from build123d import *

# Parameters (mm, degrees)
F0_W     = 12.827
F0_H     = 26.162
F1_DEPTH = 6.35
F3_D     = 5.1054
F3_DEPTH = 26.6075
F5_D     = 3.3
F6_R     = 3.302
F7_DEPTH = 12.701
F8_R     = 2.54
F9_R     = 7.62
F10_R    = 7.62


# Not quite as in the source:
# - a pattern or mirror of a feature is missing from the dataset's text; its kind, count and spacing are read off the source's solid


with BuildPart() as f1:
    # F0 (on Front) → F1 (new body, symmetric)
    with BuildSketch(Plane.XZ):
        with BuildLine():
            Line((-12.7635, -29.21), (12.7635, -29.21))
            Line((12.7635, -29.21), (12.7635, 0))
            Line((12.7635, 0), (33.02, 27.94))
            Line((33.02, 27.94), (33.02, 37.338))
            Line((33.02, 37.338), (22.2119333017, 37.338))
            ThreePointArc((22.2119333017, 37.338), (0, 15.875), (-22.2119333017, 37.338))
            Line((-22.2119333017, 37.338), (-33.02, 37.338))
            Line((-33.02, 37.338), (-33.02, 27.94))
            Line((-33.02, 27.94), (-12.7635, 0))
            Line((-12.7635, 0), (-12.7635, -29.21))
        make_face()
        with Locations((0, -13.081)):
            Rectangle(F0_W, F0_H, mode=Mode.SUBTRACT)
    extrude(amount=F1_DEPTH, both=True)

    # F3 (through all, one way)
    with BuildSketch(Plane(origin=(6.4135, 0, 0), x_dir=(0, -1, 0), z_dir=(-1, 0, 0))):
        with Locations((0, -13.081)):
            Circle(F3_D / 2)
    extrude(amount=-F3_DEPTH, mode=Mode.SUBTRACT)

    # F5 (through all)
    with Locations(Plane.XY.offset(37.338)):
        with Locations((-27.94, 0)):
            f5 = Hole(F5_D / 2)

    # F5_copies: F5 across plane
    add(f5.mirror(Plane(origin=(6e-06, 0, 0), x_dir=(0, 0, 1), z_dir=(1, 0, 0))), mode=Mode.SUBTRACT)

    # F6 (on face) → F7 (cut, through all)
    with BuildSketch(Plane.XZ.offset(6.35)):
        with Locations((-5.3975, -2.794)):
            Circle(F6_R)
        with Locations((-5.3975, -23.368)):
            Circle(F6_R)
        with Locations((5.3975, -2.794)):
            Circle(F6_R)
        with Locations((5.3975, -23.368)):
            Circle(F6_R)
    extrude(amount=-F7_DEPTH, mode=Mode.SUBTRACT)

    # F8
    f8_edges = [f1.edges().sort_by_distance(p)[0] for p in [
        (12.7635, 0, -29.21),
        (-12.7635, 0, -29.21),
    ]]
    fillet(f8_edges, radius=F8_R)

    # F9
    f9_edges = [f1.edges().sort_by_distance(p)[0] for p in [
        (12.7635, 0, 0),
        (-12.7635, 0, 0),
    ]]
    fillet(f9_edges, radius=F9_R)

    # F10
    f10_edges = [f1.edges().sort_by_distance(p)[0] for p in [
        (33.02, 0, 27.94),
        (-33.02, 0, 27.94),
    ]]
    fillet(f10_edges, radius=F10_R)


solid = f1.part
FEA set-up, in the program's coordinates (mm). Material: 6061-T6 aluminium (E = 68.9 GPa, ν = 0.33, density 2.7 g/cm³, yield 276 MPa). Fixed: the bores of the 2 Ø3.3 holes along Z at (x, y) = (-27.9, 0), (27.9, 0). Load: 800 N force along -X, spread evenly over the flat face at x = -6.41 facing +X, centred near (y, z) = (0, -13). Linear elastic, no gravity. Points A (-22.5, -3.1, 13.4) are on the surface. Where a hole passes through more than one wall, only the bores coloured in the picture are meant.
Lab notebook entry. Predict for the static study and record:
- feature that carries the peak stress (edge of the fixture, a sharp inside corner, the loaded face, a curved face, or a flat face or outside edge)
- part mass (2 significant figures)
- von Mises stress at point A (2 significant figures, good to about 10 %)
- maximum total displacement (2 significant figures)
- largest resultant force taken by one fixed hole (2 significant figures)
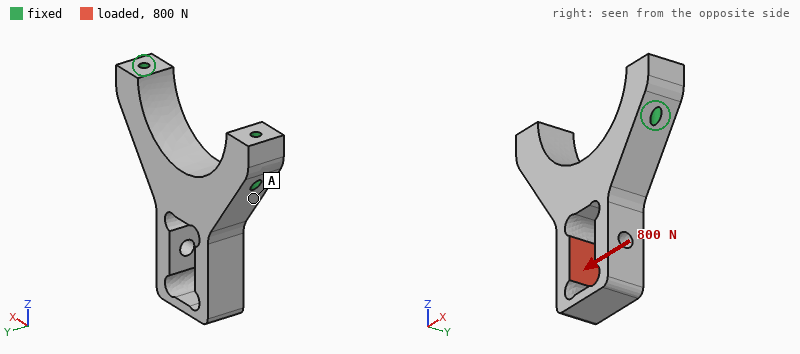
a curved face
51 g
10 MPa
95 µm
760 N
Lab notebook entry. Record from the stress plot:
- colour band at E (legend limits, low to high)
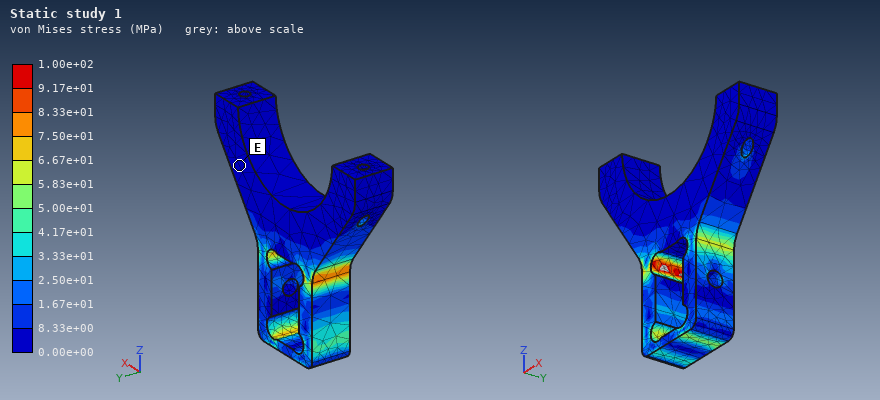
0.00e+00 to 8.33e+00 MPa
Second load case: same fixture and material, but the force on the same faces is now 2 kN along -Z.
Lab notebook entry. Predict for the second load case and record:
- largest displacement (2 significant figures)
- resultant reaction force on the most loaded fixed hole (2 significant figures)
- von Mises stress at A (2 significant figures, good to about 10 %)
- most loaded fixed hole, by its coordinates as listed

77 µm
1.5 kN
15 MPa
(-27.9, 0)
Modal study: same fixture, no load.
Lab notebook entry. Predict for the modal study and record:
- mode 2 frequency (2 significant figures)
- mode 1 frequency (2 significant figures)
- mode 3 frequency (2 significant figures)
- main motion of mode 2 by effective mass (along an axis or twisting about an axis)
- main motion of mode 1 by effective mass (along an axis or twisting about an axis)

4300 Hz
3100 Hz
8200 Hz
along X
along Y
